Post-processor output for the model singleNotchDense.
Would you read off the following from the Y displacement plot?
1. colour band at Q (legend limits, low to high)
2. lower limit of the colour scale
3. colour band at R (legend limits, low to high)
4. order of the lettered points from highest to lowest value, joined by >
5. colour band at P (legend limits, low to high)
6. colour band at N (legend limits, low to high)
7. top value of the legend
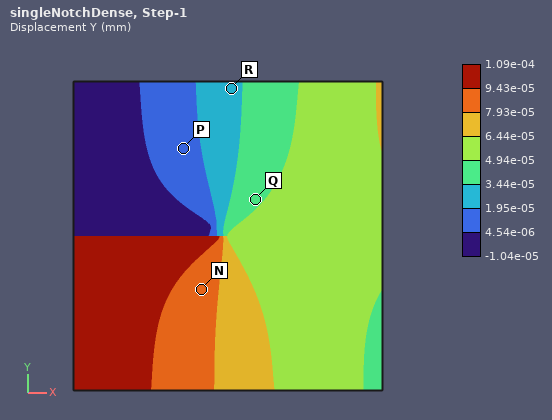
3.44e-05 to 4.94e-05 mm
-1.04e-05 mm
1.95e-05 to 3.44e-05 mm
N > Q > R > P
4.54e-06 to 1.95e-05 mm
7.93e-05 to 9.43e-05 mm
1.09e-04 mm
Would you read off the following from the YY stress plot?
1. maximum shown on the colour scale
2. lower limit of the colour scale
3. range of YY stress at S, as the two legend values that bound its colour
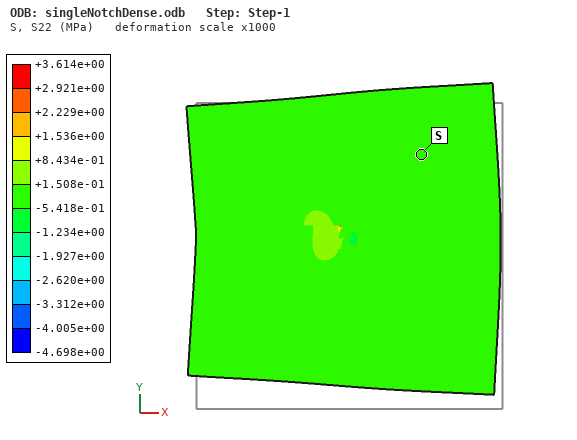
+3.614e+00 MPa
-4.698e+00 MPa
-5.418e-01 to +1.508e-01 MPa
